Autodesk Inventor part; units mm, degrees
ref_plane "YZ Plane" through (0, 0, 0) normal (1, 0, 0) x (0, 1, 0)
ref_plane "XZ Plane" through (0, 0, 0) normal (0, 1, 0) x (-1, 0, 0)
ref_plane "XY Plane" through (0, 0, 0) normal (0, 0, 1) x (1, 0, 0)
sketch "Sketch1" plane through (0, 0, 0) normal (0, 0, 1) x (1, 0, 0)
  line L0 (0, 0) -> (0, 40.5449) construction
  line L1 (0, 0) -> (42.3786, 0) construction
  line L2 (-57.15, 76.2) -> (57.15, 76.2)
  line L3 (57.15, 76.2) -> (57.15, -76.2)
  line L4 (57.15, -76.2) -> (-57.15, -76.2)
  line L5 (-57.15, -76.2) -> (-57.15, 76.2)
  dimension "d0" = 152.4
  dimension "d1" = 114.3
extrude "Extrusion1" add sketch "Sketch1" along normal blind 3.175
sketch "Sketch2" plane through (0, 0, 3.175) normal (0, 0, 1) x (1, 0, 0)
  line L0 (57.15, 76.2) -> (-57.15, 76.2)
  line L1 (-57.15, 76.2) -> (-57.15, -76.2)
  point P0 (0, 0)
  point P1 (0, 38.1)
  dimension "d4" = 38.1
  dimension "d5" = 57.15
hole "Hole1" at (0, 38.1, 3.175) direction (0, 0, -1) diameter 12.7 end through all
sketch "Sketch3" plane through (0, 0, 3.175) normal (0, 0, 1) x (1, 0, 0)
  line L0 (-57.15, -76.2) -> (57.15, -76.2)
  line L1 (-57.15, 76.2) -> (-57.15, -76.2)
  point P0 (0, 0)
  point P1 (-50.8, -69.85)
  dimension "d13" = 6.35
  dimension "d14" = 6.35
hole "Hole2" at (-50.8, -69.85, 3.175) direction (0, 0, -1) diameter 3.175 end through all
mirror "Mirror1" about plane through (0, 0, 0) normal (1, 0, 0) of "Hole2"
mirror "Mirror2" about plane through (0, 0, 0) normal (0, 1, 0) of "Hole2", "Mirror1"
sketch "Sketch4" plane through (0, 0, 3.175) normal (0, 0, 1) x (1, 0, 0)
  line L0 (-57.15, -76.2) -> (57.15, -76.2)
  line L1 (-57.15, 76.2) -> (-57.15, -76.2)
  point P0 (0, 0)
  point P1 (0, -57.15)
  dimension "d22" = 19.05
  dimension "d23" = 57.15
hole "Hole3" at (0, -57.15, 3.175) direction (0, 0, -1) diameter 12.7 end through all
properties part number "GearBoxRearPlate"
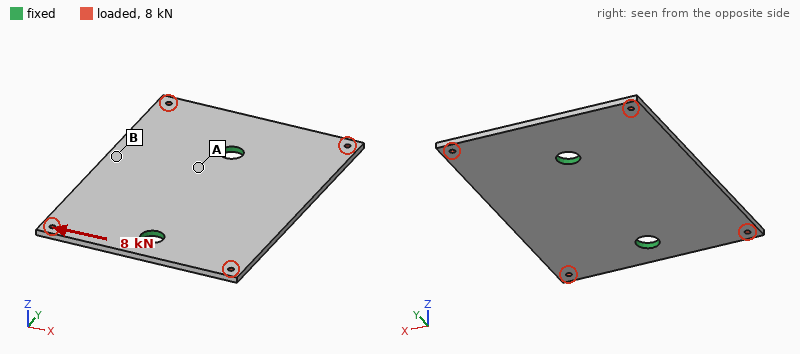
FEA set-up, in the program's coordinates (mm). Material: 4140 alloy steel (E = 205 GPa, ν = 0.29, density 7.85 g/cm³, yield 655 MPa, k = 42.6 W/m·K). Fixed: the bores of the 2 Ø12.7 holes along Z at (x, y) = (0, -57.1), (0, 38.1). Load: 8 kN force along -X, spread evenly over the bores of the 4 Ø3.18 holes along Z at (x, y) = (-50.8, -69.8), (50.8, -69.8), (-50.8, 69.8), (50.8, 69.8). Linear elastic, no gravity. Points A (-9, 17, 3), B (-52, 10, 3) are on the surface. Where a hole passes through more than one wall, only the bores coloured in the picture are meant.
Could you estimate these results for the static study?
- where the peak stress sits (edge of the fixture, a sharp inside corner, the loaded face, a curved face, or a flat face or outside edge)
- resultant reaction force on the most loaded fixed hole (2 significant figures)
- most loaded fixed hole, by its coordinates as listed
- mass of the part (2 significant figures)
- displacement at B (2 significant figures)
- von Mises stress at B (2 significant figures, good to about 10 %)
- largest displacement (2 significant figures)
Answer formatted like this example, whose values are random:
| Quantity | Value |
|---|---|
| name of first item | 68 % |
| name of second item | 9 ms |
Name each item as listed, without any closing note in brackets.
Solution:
| Quantity | Value |
|---|---|
| where the peak stress sits | the loaded face |
| resultant reaction force on the most loaded fixed hole | 4.7 kN |
| most loaded fixed hole, by its coordinates as listed | (0, 38.1) |
| mass of the part | 430 g |
| displacement at B | 2.5 µm |
| von Mises stress at B | 16 MPa |
| largest displacement | 17 µm |
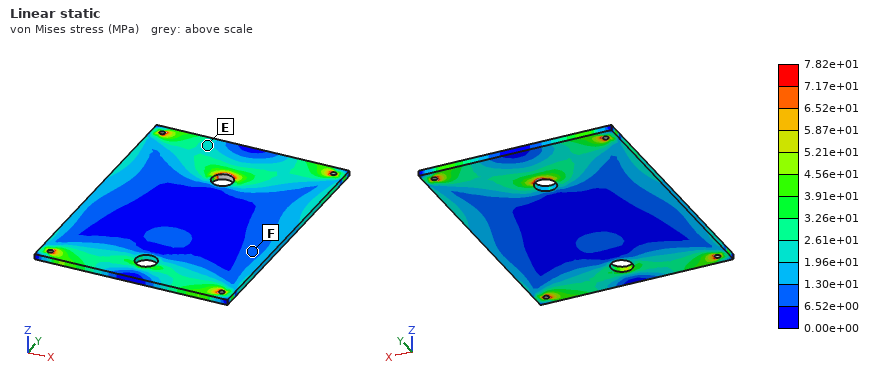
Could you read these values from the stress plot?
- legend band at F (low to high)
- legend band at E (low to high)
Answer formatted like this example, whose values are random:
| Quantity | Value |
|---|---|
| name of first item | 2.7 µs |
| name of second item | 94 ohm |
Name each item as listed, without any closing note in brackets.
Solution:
| Quantity | Value |
|---|---|
| legend band at F | 6.52e+00 to 1.30e+01 MPa |
| legend band at E | 1.96e+01 to 2.61e+01 MPa |
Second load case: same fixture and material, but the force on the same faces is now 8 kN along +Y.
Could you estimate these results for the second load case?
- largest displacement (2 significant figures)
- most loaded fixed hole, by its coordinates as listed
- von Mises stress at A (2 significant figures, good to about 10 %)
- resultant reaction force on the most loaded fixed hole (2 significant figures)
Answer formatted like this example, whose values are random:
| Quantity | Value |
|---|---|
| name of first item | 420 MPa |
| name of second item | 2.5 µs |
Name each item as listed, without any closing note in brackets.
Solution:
| Quantity | Value |
|---|---|
| largest displacement | 15 µm |
| most loaded fixed hole, by its coordinates as listed | (0, 38.1) |
| von Mises stress at A | 21 MPa |
| resultant reaction force on the most loaded fixed hole | 4.6 kN |
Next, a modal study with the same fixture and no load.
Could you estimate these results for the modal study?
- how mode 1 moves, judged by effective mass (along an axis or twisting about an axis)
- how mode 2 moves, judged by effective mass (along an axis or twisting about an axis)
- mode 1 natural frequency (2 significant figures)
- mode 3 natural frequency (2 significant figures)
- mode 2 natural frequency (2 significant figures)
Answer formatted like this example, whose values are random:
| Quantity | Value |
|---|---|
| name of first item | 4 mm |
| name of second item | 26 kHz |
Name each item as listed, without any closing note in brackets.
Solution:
| Quantity | Value |
|---|---|
| how mode 1 moves, judged by effective mass | twisting about Y |
| how mode 2 moves, judged by effective mass | along Z |
| mode 1 natural frequency | 730 Hz |
| mode 3 natural frequency | 1000 Hz |
| mode 2 natural frequency | 870 Hz |
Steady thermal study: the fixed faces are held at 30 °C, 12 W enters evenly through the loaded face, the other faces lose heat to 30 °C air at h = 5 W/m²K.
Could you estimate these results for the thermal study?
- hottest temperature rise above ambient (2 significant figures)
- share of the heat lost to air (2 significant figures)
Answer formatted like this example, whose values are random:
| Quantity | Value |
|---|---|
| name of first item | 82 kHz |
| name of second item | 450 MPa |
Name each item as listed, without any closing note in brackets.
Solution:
| Quantity | Value |
|---|---|
| hottest temperature rise above ambient | 36 K |
| share of the heat lost to air | 17 % |
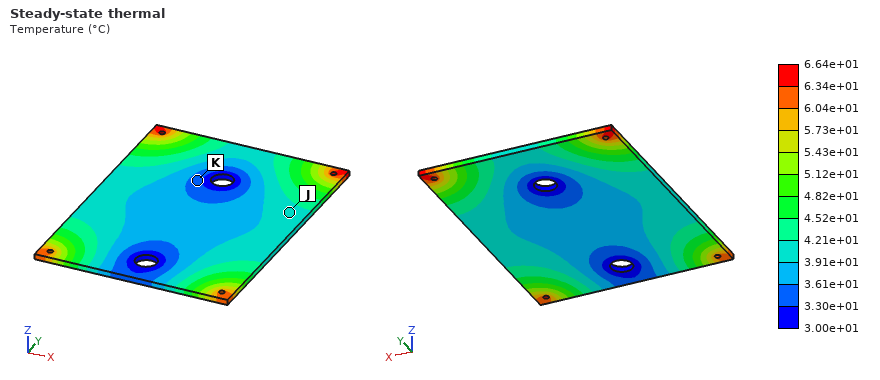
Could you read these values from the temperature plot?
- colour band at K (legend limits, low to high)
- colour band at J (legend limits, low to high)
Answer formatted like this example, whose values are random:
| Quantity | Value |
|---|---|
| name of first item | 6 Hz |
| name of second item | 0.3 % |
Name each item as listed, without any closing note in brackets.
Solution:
| Quantity | Value |
|---|---|
| colour band at K | 3.30e+01 to 3.61e+01 °C |
| colour band at J | 3.91e+01 to 4.21e+01 °C |
